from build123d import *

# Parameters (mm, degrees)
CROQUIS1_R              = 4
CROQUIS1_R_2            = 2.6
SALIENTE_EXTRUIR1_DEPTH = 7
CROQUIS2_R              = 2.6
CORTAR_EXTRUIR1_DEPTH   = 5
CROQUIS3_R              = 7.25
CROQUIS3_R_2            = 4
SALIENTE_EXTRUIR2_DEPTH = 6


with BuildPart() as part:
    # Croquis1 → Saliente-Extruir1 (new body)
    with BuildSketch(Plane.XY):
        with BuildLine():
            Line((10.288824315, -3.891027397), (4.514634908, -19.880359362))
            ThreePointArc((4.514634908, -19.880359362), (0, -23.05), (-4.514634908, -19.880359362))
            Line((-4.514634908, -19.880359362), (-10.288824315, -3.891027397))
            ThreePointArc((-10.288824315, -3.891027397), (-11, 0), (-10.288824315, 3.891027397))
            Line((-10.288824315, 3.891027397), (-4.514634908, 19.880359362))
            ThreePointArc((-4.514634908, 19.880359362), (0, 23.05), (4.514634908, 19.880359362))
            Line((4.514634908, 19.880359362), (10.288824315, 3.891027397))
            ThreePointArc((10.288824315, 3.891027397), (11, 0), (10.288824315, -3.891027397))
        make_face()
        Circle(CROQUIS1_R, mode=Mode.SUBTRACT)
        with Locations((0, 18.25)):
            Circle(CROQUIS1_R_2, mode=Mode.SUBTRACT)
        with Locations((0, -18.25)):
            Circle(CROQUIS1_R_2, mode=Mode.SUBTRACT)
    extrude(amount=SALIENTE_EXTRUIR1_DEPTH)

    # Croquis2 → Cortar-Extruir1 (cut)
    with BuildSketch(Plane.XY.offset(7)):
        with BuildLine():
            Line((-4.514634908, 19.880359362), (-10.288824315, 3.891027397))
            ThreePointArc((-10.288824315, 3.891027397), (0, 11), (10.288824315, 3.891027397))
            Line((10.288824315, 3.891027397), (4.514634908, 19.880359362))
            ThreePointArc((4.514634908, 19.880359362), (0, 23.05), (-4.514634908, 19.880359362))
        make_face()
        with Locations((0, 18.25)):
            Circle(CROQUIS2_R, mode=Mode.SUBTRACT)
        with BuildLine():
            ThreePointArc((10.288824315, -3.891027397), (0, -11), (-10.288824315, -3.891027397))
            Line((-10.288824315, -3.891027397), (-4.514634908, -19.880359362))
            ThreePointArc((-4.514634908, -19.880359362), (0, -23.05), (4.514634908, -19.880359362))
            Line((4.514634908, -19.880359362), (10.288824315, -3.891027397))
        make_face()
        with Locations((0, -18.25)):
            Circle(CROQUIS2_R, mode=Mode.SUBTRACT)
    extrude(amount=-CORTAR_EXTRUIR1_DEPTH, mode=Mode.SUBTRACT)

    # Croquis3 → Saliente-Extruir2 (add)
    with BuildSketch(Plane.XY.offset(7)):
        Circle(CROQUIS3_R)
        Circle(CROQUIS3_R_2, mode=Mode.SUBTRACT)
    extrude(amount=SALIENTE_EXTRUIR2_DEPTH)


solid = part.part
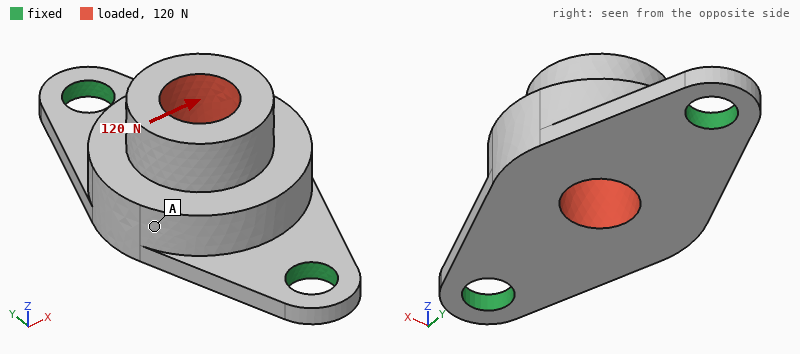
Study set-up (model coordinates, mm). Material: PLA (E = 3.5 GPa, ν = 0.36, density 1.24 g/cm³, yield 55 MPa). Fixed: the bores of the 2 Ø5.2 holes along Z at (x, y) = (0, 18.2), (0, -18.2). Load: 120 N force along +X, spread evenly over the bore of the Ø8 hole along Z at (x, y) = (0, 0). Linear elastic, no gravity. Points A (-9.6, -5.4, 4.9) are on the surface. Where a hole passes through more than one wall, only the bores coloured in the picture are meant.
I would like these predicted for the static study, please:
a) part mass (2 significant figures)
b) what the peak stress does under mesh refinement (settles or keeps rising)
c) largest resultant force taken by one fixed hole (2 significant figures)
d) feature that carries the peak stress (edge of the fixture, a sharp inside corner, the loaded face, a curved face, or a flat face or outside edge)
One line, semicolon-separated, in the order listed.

4.4 g; keeps rising; 60 N; edge of the fixture
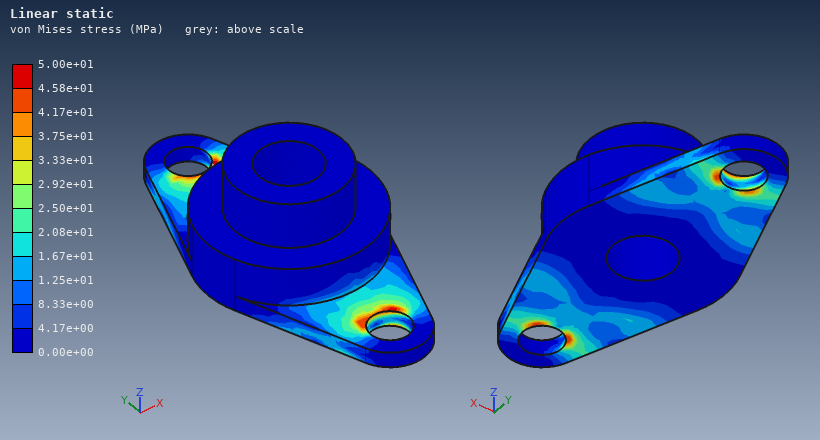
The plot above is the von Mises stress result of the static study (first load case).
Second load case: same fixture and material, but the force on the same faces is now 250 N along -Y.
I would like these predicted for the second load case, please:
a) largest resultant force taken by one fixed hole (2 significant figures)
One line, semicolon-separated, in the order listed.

130 N
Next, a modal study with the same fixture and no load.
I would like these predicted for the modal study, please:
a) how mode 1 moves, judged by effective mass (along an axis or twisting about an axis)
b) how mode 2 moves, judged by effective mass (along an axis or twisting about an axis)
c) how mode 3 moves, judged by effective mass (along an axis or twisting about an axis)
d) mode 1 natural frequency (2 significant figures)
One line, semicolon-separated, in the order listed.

along X; along Z; along Y; 1500 Hz
